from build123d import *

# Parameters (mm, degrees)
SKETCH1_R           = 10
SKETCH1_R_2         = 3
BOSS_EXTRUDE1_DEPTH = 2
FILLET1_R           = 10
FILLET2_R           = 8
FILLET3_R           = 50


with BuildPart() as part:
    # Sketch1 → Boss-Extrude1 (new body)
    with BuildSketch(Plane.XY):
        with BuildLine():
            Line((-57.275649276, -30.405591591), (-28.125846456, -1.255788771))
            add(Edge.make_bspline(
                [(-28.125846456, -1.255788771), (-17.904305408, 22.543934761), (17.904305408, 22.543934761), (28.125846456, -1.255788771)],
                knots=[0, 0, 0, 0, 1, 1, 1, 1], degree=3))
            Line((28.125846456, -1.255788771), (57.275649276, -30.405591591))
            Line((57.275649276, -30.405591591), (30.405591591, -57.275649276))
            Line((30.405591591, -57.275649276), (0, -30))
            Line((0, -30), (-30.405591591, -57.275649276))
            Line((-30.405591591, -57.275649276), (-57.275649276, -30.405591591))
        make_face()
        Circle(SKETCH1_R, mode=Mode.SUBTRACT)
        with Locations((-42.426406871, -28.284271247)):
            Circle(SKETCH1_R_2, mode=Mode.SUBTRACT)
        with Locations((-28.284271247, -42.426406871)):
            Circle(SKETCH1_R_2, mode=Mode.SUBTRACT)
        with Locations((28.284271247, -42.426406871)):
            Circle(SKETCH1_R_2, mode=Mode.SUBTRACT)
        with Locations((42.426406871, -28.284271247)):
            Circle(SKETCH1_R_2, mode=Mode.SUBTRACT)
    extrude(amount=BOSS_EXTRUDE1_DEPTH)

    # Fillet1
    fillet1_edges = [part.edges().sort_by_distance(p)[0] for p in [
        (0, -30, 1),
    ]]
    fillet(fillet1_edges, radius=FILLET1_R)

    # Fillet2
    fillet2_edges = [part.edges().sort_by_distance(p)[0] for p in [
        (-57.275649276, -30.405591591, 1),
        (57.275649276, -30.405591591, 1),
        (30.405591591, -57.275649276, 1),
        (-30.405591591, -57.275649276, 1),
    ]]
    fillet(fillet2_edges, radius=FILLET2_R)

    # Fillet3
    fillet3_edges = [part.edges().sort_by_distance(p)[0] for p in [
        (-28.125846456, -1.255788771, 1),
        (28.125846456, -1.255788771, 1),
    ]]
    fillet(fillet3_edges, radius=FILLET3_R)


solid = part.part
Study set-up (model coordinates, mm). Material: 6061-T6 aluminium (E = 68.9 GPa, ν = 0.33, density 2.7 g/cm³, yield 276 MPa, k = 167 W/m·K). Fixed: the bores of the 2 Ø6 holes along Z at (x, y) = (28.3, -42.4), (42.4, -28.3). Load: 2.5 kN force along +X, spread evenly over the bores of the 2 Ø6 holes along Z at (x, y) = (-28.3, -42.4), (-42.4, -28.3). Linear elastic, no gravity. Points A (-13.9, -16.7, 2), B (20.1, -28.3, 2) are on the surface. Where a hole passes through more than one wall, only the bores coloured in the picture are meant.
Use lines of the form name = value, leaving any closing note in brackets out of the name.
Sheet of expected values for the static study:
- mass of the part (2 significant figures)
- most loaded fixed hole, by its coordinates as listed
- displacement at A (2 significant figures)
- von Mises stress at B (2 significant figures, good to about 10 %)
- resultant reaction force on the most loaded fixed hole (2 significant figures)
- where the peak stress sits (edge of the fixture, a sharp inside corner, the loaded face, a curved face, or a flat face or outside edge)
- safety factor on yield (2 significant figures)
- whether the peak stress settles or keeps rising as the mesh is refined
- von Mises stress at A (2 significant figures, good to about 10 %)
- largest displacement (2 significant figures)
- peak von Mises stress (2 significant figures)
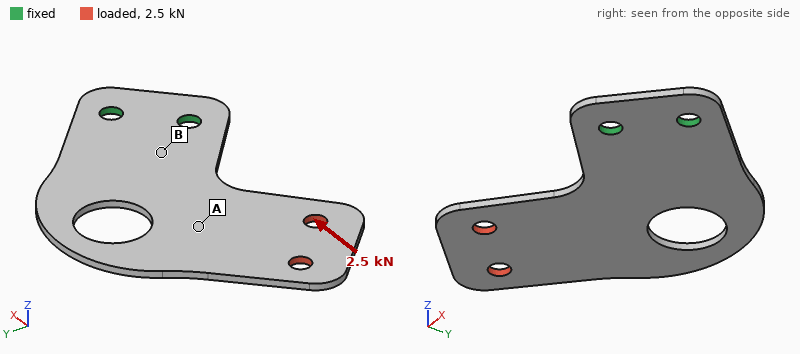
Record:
mass of the part = 23 g
most loaded fixed hole, by its coordinates as listed = (28.3, -42.4)
displacement at A = 0.045 mm
von Mises stress at B = 57 MPa
resultant reaction force on the most loaded fixed hole = 1.3 kN
where the peak stress sits = a curved face
safety factor on yield = 1.0
whether the peak stress settles or keeps rising as the mesh is refined = settles
von Mises stress at A = 24 MPa
largest displacement = 0.21 mm
peak von Mises stress = 260 MPa
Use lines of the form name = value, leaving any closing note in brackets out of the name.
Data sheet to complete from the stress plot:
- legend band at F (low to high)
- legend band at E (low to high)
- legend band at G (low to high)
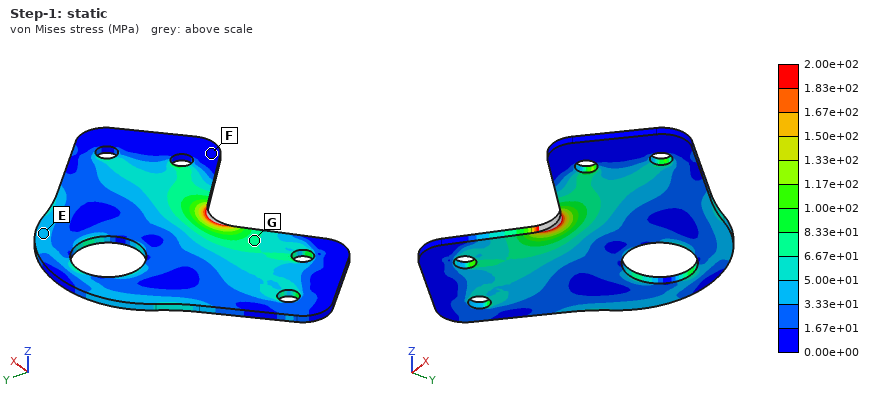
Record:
legend band at F = 0.00e+00 to 1.67e+01 MPa
legend band at E = 3.33e+01 to 5.00e+01 MPa
legend band at G = 6.67e+01 to 8.33e+01 MPa
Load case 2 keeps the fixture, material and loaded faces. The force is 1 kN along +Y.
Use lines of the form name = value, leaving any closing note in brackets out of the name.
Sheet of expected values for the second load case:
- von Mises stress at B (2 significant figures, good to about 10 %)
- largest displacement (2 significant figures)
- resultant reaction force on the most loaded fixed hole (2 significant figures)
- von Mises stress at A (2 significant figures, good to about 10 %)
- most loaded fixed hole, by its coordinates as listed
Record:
von Mises stress at B = 45 MPa
largest displacement = 0.39 mm
resultant reaction force on the most loaded fixed hole = 3.3 kN
von Mises stress at A = 32 MPa
most loaded fixed hole, by its coordinates as listed = (28.3, -42.4)
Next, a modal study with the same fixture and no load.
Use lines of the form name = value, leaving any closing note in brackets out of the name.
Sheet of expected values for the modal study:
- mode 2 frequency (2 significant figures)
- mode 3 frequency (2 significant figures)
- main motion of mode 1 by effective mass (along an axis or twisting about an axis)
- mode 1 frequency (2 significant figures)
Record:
mode 2 frequency = 560 Hz
mode 3 frequency = 1500 Hz
main motion of mode 1 by effective mass = along Z
mode 1 frequency = 230 Hz
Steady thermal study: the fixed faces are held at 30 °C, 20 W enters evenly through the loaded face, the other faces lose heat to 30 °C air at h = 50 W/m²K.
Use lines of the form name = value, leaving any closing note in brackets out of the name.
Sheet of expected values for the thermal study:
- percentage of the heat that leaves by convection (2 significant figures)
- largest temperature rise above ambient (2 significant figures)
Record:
percentage of the heat that leaves by convection = 64 %
largest temperature rise above ambient = 70 K
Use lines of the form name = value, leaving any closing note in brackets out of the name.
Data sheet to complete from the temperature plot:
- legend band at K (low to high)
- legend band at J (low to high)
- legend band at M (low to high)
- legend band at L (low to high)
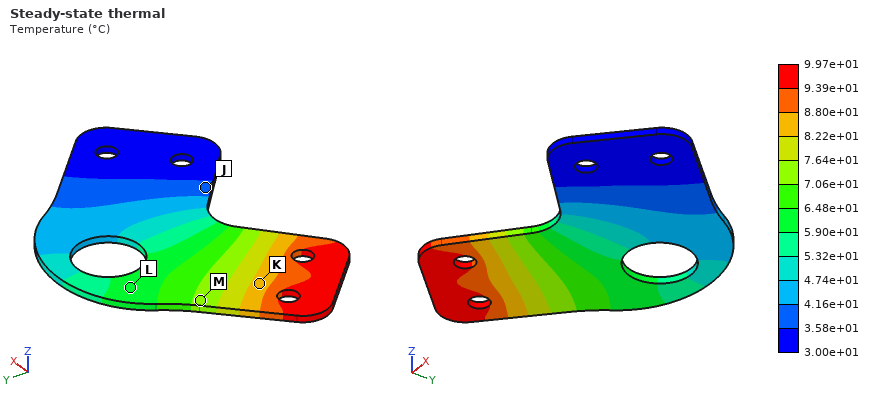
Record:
legend band at K = 8.22e+01 to 8.80e+01 °C
legend band at J = 3.58e+01 to 4.16e+01 °C
legend band at M = 7.06e+01 to 7.64e+01 °C
legend band at L = 5.90e+01 to 6.48e+01 °C
